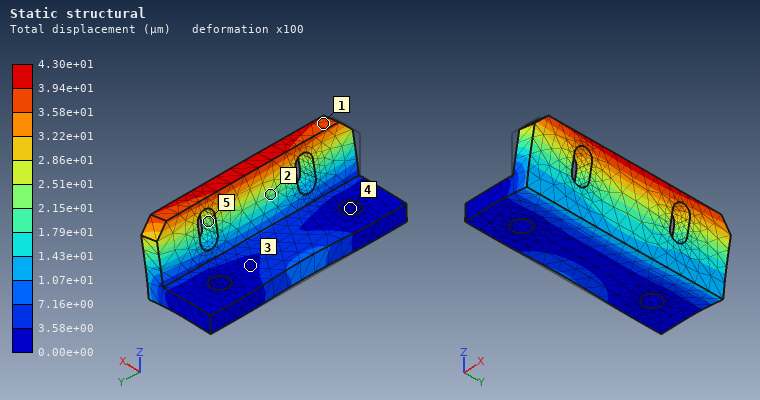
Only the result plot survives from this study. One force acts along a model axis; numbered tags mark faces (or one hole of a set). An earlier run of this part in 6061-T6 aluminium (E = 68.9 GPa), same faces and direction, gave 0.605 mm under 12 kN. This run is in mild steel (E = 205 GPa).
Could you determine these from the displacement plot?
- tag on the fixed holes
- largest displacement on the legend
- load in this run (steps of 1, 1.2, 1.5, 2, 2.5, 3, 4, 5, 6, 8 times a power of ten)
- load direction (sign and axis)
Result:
4
4.30e+01 µm
2.5 kN
+X
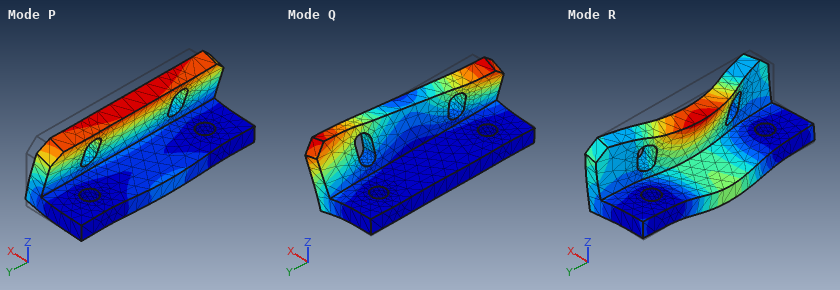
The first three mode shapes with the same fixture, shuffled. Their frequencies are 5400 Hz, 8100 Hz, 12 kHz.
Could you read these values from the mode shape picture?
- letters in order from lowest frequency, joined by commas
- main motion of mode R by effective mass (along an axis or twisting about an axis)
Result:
P, Q, R
along Z
